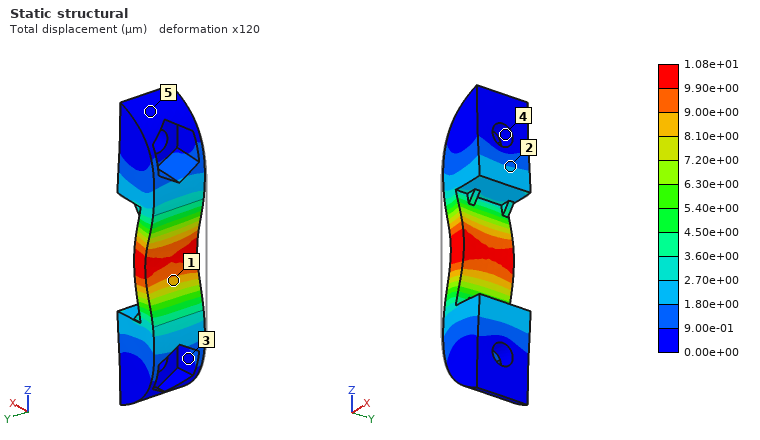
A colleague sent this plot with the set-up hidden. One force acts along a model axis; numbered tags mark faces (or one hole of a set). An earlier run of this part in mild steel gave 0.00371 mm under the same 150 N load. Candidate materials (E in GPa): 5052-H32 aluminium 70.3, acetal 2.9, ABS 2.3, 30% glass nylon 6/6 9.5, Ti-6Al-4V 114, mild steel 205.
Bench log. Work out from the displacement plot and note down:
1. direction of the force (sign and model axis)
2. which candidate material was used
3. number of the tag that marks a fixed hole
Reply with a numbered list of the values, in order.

1. +X
2. 5052-H32 aluminium
3. 4
